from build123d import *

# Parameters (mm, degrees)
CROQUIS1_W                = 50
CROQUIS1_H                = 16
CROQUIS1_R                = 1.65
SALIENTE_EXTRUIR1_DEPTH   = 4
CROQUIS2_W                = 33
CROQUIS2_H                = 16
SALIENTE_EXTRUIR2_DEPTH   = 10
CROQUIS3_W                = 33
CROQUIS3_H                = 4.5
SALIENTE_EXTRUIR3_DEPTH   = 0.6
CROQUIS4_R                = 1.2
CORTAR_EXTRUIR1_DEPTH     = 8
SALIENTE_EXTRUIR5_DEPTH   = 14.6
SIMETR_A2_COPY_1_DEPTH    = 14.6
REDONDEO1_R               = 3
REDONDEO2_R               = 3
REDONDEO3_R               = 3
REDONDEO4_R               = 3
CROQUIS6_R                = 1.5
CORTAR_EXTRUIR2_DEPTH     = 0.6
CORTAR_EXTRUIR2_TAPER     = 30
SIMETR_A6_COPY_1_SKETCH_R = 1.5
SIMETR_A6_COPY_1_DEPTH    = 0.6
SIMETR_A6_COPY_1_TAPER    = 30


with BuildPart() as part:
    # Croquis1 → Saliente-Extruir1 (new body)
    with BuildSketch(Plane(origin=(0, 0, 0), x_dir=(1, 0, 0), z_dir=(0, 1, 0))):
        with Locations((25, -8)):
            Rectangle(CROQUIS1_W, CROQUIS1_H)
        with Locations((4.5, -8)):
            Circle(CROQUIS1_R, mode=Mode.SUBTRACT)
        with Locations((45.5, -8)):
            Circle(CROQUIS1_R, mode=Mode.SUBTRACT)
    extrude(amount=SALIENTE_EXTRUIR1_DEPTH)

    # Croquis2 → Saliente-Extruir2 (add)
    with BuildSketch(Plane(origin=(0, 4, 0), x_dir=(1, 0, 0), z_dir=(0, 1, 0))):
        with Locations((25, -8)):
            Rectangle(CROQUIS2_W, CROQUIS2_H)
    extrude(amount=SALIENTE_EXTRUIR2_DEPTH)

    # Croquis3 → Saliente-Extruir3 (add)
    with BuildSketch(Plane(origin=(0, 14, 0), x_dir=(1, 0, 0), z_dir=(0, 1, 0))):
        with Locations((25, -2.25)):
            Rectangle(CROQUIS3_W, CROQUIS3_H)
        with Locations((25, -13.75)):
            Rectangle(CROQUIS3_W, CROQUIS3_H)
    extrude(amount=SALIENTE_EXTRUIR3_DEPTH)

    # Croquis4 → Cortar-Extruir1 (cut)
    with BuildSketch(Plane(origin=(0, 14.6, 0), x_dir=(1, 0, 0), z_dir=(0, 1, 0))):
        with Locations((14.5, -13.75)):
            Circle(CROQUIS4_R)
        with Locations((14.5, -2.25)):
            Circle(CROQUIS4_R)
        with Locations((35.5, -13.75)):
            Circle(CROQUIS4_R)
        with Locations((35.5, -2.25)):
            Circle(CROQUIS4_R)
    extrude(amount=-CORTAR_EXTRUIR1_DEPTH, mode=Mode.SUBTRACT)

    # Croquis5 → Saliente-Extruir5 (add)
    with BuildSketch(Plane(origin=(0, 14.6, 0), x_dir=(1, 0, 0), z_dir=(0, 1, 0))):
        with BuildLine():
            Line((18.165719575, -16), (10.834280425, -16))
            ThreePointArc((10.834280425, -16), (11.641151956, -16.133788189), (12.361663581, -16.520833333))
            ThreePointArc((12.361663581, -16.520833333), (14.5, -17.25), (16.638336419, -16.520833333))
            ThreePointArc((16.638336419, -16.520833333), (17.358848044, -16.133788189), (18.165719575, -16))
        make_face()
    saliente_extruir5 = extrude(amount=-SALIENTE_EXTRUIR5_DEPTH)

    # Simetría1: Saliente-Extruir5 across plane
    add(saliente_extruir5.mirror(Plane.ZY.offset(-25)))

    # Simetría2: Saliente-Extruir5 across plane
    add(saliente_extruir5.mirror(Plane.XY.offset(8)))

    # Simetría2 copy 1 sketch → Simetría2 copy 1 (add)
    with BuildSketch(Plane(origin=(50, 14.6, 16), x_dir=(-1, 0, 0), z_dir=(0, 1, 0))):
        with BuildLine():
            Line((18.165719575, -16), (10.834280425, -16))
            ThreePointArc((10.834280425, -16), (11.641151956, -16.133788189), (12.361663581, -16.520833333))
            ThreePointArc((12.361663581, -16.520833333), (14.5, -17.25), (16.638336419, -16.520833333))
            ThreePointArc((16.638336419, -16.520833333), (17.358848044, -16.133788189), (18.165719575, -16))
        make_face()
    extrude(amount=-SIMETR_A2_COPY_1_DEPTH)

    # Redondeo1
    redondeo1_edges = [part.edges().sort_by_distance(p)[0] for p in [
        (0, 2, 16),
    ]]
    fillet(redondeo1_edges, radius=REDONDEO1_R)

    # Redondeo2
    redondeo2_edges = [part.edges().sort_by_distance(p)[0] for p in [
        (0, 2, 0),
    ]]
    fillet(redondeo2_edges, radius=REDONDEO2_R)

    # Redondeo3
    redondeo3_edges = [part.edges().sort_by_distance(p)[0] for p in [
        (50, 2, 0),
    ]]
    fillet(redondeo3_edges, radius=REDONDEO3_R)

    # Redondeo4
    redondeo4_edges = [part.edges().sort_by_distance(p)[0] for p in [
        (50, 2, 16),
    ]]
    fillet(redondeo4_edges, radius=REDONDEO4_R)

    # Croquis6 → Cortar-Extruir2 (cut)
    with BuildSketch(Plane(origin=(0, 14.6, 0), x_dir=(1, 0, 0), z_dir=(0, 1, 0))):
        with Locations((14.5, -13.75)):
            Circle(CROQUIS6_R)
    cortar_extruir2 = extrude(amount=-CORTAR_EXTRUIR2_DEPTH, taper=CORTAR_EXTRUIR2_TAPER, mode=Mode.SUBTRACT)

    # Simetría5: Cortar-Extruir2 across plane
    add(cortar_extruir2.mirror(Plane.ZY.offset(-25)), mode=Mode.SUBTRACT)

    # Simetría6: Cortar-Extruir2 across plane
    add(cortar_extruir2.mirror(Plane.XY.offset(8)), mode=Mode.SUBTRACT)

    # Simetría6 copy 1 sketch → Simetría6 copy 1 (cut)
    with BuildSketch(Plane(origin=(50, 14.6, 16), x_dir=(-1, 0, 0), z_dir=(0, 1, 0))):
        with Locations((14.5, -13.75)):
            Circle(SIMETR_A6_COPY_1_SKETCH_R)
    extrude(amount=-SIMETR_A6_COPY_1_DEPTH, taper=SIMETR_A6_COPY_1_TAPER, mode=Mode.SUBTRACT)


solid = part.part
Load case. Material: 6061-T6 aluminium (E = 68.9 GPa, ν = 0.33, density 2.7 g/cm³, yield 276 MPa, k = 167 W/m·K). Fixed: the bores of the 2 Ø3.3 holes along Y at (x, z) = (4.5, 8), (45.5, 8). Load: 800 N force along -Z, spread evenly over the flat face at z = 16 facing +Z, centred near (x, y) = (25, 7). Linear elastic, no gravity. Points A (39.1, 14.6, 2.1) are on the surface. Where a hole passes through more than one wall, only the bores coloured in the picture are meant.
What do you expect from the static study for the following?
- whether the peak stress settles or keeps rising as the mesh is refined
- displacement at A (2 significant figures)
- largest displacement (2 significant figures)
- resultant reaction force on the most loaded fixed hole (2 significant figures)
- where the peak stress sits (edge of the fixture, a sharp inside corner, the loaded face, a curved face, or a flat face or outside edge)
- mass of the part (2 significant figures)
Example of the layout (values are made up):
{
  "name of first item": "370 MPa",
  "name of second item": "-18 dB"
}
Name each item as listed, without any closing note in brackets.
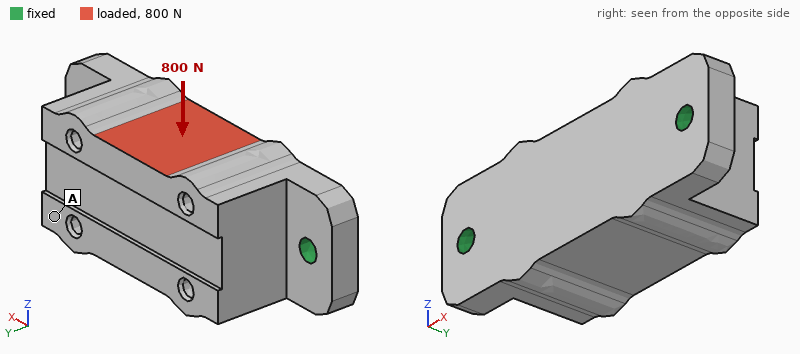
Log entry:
{
  "whether the peak stress settles or keeps rising as the mesh is refined": "keeps rising",
  "displacement at A": "21 µm",
  "largest displacement": "25 µm",
  "resultant reaction force on the most loaded fixed hole": "400 N",
  "where the peak stress sits": "edge of the fixture",
  "mass of the part": "23 g"
}
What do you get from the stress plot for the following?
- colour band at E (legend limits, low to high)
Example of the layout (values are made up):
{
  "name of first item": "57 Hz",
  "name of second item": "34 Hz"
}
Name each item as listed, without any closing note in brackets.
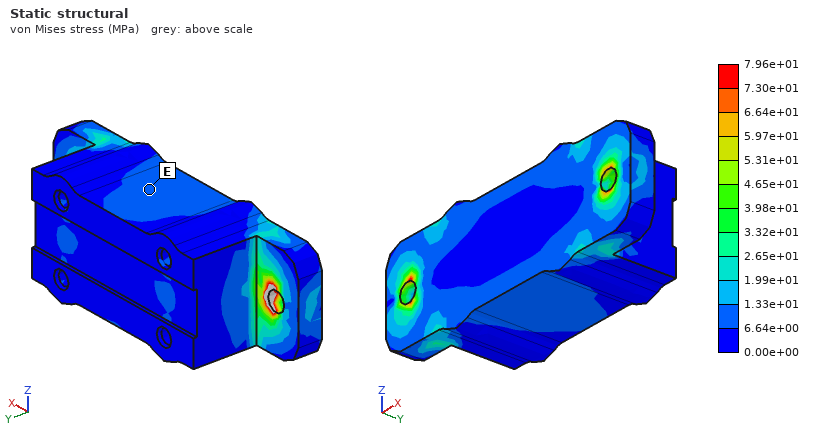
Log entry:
{
  "colour band at E": "6.64e+00 to 1.33e+01 MPa"
}
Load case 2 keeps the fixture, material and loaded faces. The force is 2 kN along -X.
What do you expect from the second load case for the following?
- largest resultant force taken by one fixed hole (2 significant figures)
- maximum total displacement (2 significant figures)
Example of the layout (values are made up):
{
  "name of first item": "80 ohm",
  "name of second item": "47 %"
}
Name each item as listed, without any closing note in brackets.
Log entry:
{
  "largest resultant force taken by one fixed hole": "1.1 kN",
  "maximum total displacement": "7.2 µm"
}
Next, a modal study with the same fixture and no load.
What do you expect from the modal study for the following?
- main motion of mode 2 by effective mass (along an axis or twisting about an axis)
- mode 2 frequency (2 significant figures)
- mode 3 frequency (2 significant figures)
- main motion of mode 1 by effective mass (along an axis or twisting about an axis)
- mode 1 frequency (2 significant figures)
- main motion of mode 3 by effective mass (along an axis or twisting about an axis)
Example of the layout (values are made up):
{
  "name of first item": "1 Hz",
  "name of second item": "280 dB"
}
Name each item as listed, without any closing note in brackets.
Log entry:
{
  "main motion of mode 2 by effective mass": "along Y",
  "mode 2 frequency": "15 kHz",
  "mode 3 frequency": "21 kHz",
  "main motion of mode 1 by effective mass": "along Z",
  "mode 1 frequency": "7300 Hz",
  "main motion of mode 3 by effective mass": "along Z"
}
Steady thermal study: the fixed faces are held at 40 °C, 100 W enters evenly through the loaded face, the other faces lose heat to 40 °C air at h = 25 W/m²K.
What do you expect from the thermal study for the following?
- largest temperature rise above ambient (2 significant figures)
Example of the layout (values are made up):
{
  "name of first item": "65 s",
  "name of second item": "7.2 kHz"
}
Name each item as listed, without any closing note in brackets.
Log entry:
{
  "largest temperature rise above ambient": "64 K"
}
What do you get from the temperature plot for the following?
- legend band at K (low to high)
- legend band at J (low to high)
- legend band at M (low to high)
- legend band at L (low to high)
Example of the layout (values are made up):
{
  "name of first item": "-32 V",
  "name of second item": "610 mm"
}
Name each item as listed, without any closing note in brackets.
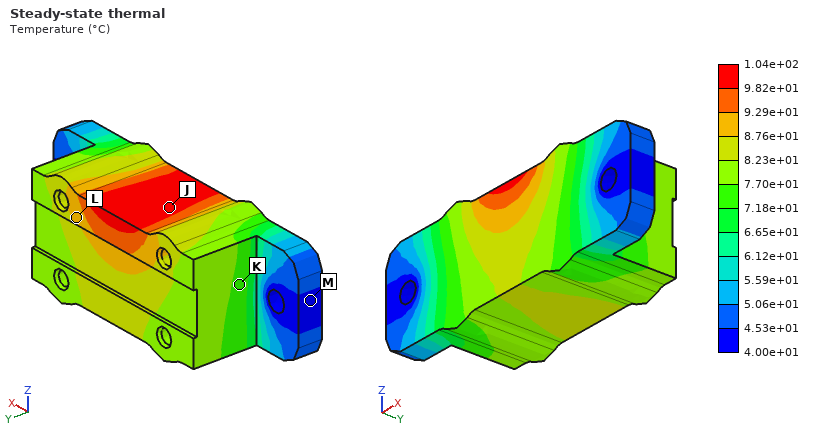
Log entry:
{
  "legend band at K": "7.18e+01 to 7.70e+01 °C",
  "legend band at J": "9.82e+01 to 1.04e+02 °C",
  "legend band at M": "4.00e+01 to 4.53e+01 °C",
  "legend band at L": "8.76e+01 to 9.29e+01 °C"
}
